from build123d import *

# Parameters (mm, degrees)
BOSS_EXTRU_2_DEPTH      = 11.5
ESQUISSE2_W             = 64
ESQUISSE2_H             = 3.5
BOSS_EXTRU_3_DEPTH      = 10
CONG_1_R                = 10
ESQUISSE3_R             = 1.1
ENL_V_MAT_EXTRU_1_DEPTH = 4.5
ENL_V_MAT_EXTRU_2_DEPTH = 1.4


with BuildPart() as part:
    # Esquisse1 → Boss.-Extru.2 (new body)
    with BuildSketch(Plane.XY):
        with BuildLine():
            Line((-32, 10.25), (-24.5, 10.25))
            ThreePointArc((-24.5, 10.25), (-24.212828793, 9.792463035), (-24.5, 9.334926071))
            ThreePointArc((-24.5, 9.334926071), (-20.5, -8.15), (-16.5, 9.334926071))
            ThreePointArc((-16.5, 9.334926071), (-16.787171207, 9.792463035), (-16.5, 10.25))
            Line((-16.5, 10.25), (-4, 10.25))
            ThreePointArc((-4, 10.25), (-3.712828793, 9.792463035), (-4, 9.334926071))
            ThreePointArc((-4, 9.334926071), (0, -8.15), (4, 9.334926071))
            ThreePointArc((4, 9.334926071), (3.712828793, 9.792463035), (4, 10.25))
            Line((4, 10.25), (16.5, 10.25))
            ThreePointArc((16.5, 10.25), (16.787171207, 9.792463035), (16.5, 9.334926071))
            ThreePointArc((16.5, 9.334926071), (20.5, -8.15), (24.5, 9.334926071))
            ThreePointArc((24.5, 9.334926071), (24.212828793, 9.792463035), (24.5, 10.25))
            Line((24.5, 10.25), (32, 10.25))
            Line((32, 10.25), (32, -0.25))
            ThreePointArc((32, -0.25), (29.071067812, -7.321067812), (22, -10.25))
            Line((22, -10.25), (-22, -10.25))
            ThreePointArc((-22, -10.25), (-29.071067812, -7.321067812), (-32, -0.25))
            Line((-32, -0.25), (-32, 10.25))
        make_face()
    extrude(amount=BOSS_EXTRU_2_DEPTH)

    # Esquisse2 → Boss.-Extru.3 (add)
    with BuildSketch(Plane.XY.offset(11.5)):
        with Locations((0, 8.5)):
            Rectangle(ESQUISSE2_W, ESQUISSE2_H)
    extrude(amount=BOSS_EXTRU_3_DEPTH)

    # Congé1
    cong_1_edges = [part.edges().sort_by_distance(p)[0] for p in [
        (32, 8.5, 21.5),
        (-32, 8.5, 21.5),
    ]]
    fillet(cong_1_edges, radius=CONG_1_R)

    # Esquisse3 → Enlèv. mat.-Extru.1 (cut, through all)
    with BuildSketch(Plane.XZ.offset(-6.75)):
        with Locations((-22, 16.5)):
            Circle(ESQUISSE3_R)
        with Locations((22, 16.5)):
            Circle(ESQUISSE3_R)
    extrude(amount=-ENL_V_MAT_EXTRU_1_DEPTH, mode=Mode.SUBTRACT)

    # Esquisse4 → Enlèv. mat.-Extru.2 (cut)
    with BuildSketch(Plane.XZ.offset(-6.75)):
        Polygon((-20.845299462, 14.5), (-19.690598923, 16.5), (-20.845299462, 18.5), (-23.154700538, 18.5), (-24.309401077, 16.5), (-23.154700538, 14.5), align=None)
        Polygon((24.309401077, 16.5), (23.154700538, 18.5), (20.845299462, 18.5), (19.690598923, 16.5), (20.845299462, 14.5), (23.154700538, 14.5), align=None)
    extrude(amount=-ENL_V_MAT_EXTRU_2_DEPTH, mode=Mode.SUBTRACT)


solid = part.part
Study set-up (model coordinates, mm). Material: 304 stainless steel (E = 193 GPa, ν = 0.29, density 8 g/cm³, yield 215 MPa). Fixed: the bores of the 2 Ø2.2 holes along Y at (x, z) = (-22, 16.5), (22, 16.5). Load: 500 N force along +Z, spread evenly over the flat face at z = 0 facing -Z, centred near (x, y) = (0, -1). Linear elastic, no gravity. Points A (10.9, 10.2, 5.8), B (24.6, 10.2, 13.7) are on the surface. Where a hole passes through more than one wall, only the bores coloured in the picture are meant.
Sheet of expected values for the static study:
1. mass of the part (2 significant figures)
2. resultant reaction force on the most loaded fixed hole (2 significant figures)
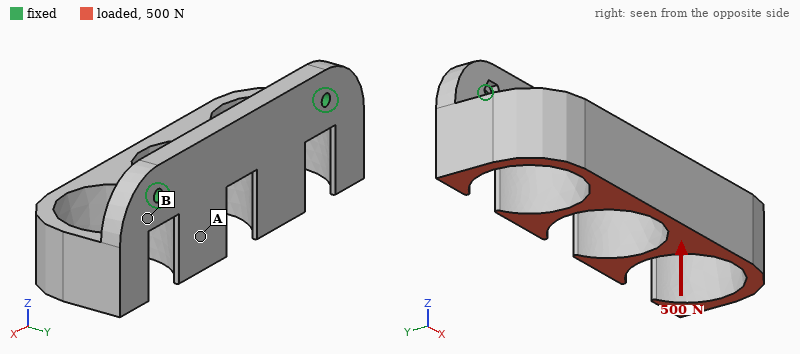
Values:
59 g
250 N
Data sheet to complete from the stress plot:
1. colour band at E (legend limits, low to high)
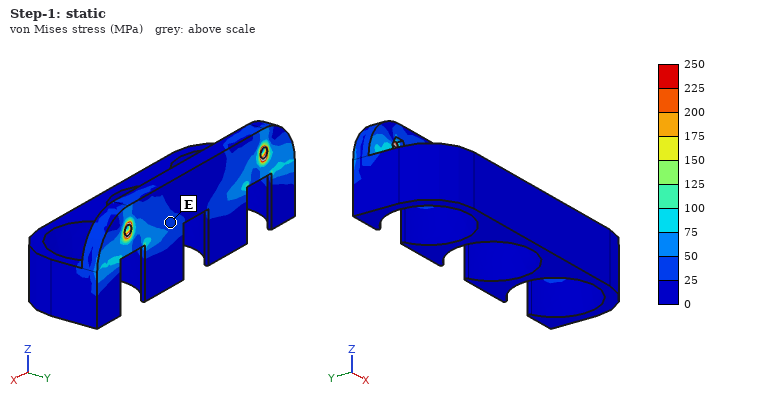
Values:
25 to 50 MPa
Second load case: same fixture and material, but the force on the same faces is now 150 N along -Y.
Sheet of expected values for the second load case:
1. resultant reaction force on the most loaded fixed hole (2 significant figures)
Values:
77 N
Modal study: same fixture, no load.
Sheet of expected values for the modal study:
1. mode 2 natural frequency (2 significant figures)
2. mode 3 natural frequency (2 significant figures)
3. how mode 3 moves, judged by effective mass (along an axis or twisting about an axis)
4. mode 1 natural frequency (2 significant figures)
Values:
3800 Hz
6000 Hz
along X
1800 Hz
